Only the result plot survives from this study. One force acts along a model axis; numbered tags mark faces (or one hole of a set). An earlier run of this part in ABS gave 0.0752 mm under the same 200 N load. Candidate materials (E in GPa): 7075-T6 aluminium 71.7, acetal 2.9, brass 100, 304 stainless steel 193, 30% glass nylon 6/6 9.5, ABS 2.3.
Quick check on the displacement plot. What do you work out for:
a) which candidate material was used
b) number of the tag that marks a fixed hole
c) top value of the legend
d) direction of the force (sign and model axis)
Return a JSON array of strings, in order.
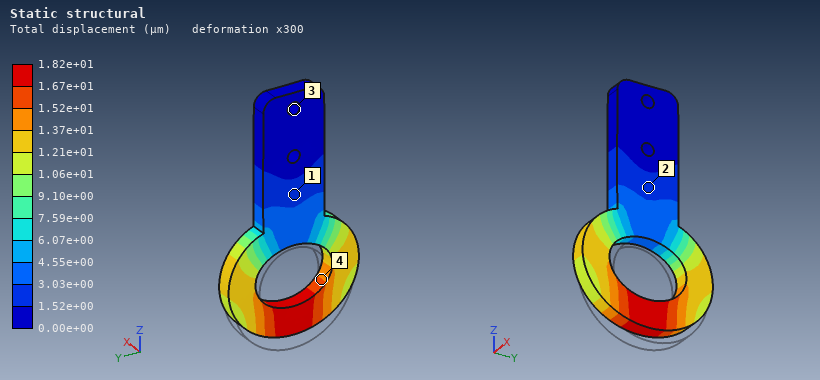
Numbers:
["30% glass nylon 6/6", "3", "1.82e+01 µm", "+Z"]
